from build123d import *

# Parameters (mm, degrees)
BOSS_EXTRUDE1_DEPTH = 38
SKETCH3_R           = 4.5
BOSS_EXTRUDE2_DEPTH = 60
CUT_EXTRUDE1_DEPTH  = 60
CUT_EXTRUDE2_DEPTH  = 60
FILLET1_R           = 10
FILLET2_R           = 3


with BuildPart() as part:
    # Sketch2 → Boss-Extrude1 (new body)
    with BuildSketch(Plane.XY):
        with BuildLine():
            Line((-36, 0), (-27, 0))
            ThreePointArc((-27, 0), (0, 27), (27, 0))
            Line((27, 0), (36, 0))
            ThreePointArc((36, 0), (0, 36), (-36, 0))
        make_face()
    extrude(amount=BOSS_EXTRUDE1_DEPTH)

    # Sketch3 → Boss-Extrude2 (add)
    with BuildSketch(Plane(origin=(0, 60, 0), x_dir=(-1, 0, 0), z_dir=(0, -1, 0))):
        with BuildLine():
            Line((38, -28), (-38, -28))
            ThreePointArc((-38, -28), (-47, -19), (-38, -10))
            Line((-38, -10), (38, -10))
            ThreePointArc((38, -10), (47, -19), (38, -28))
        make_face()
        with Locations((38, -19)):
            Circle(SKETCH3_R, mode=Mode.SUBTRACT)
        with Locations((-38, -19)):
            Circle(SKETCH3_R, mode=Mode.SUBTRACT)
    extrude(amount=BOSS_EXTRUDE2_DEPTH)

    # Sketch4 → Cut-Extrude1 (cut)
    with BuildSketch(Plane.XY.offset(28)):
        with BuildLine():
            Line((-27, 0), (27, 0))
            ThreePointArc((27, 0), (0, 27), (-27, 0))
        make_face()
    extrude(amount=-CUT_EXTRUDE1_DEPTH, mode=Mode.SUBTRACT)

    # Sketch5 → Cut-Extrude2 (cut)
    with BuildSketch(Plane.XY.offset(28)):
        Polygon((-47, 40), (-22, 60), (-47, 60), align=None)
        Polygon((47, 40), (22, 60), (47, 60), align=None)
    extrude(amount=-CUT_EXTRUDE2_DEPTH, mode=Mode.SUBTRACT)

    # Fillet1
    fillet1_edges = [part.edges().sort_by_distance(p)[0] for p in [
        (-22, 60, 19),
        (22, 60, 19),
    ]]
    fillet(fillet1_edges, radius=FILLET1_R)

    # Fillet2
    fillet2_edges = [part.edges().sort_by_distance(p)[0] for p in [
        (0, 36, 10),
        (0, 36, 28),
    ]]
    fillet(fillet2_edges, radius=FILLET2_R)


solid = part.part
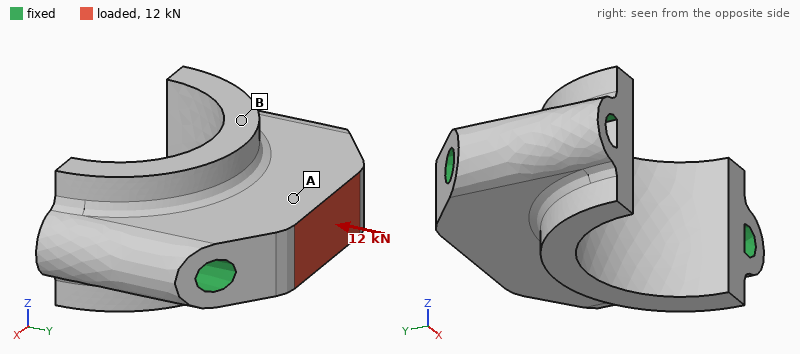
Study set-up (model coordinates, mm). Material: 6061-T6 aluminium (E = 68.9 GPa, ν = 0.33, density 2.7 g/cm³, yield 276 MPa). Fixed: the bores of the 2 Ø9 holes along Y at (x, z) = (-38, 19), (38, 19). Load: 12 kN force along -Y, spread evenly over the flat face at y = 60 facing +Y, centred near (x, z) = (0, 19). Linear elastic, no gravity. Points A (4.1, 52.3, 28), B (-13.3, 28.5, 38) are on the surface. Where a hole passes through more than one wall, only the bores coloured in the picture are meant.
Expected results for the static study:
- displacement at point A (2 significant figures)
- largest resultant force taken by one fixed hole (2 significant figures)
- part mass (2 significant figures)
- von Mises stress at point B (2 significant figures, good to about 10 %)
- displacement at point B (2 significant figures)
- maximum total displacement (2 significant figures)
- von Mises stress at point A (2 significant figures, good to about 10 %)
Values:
12 µm
7.0 kN
220 g
5.0 MPa
5.8 µm
14 µm
15 MPa
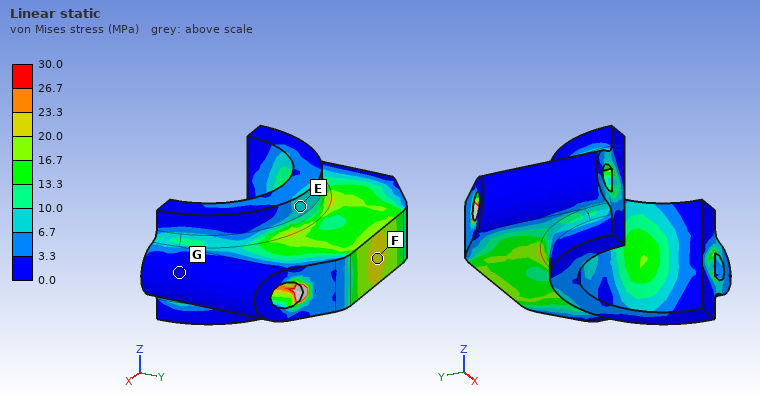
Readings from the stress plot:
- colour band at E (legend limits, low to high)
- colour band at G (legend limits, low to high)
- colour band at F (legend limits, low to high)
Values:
6.7 to 10.0 MPa
0.0 to 3.3 MPa
20.0 to 23.3 MPa
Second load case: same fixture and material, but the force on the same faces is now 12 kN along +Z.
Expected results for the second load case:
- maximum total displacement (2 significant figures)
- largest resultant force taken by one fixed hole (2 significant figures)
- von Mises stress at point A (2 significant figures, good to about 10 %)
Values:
94 µm
6.0 kN
65 MPa
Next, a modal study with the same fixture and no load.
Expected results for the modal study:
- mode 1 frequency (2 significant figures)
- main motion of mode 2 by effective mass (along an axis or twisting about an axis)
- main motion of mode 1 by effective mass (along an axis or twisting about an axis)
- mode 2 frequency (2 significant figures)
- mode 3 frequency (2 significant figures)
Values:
12 kHz
along Y
along Z
18 kHz
19 kHz
